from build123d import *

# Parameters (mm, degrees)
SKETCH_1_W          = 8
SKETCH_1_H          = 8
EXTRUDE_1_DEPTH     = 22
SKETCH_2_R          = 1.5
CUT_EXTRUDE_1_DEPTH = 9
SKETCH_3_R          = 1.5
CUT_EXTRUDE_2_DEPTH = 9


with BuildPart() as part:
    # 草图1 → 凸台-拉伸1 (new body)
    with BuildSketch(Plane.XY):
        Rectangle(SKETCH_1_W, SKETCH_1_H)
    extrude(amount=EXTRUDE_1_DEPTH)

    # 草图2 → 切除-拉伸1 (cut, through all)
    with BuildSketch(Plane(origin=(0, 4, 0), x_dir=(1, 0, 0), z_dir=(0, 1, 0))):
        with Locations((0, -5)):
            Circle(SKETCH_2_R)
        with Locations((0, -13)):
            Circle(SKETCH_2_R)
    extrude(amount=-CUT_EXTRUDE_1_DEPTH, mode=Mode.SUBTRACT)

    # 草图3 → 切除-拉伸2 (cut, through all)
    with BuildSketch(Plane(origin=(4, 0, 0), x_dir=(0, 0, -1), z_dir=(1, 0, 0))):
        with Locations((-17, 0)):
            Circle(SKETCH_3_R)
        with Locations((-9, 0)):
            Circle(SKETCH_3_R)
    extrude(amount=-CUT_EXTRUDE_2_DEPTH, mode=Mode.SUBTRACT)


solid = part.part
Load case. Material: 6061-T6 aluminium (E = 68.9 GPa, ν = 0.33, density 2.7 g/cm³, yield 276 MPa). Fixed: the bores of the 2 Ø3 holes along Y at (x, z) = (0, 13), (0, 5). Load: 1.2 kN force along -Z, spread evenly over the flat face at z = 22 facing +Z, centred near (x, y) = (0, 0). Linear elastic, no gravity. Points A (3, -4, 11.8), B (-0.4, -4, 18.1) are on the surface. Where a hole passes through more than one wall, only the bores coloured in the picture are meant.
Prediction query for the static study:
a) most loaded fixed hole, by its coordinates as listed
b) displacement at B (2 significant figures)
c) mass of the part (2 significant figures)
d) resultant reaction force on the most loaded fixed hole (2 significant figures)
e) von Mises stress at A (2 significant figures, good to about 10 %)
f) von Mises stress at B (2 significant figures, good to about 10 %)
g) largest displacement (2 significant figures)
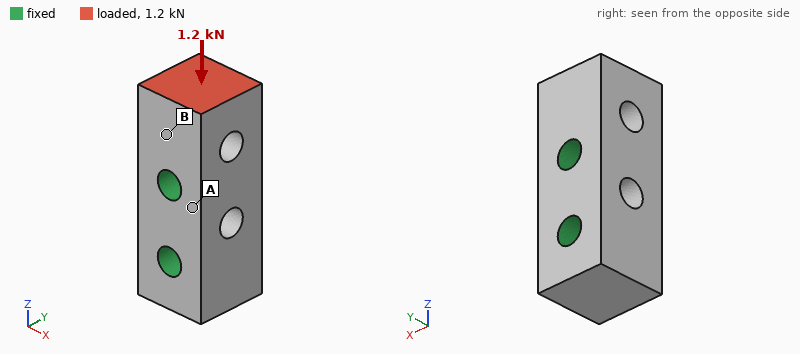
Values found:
(0, 13)
1.8 µm
3.2 g
1.1 kN
11 MPa
23 MPa
3.6 µm
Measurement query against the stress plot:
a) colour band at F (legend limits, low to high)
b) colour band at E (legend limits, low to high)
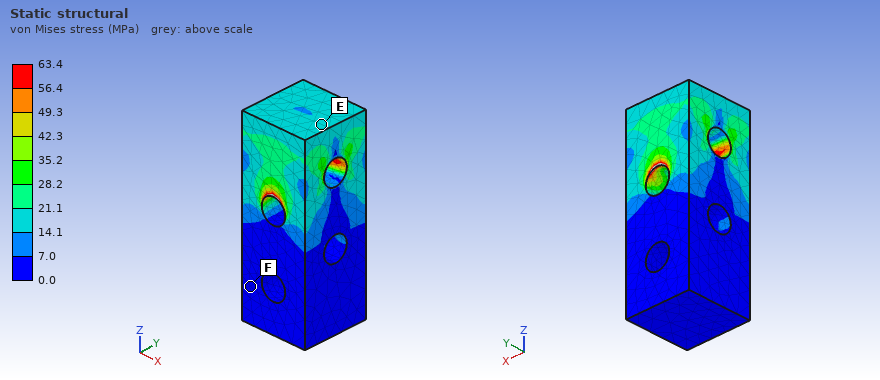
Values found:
0.0 to 7.0 MPa
14.1 to 21.1 MPa
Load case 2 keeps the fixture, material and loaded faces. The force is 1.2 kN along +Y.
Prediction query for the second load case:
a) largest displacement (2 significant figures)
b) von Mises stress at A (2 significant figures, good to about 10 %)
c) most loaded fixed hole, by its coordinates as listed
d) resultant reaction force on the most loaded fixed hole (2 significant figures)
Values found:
26 µm
40 MPa
(0, 13)
1.3 kN
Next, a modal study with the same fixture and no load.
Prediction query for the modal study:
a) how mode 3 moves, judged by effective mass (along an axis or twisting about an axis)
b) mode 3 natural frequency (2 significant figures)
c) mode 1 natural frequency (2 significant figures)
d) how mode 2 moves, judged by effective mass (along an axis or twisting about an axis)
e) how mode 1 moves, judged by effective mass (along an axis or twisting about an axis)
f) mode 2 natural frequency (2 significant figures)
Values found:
twisting about Z
74 kHz
45 kHz
along Y
along X
51 kHz
